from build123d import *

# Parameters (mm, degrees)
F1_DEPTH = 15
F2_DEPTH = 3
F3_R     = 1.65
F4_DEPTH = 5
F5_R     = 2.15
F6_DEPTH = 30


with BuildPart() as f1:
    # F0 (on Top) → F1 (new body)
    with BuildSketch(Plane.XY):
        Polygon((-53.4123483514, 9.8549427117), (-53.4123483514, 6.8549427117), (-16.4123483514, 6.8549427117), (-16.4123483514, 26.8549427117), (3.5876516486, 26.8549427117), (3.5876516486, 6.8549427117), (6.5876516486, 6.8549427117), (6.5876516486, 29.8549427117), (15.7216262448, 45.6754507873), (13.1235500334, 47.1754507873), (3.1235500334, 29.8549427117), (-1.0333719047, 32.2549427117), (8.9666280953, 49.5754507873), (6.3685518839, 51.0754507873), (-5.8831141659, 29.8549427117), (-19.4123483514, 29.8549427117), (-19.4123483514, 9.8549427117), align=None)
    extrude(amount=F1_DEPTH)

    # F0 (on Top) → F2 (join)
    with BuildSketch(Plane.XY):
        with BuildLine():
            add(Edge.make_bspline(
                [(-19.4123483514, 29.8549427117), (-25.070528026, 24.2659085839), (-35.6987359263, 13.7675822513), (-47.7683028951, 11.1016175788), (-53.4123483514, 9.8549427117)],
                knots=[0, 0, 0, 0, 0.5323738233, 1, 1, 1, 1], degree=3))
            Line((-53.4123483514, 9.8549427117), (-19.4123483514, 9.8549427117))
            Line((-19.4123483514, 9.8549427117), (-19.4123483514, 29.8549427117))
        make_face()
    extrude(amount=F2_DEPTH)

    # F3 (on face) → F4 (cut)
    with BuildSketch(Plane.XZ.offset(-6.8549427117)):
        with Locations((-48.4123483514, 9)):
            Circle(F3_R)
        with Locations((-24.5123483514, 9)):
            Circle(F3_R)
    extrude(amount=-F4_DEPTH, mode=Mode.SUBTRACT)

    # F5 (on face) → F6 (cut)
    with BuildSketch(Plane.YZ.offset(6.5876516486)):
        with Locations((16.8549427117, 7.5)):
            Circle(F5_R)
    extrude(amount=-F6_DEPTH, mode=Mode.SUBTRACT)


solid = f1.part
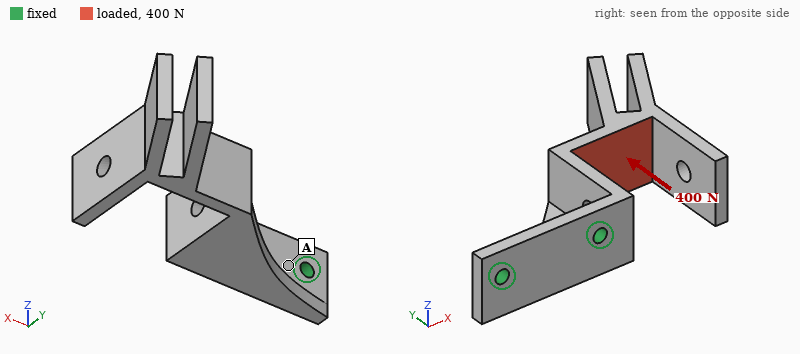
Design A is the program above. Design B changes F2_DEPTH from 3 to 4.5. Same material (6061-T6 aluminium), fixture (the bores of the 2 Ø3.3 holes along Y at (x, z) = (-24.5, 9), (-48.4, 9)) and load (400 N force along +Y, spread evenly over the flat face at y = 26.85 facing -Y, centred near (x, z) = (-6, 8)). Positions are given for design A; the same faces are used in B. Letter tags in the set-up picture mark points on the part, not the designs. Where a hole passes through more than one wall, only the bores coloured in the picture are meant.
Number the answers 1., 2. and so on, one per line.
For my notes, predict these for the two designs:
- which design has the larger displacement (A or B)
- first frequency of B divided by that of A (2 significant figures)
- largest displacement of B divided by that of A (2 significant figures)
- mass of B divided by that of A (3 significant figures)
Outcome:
1. A
2. 1.1
3. 0.86
4. 1.05
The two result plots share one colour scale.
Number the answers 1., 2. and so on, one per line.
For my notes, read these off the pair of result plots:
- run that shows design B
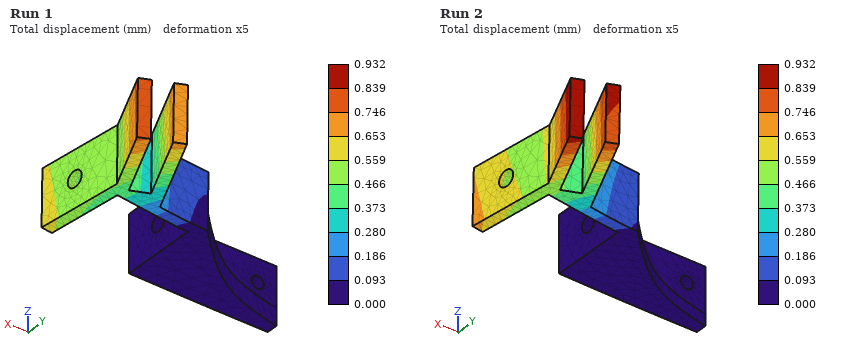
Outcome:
1. Run 1
